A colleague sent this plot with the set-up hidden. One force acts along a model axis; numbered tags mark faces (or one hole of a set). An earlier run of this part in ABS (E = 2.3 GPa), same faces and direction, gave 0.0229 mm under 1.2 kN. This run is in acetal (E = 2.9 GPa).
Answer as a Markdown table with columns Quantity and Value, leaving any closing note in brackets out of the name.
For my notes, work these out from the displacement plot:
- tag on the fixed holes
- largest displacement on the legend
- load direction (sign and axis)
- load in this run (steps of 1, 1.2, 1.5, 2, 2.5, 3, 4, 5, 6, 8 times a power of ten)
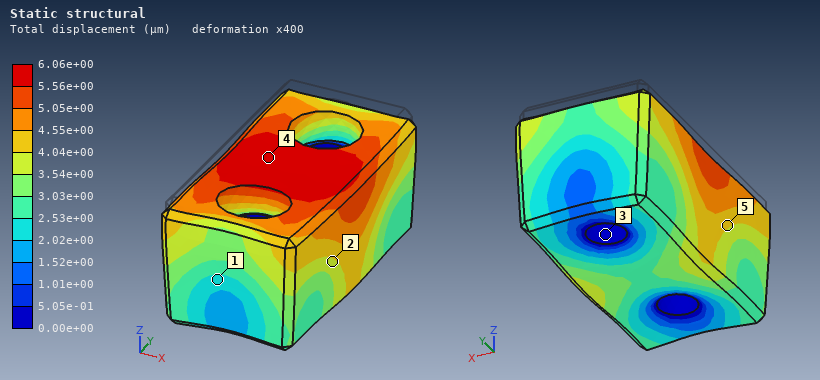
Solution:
| Quantity | Value |
|---|---|
| tag on the fixed holes | 3 |
| largest displacement on the legend | 6.06e+00 µm |
| load direction | -Z |
| load in this run | 400 N |
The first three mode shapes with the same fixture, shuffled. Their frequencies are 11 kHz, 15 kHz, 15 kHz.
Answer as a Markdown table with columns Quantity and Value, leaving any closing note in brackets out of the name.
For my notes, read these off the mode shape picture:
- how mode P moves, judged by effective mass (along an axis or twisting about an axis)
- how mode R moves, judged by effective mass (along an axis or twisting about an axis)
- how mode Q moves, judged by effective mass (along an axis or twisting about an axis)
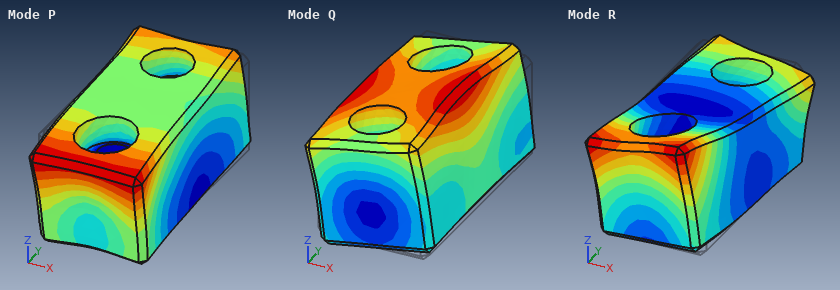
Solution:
| Quantity | Value |
|---|---|
| how mode P moves, judged by effective mass | along Y |
| how mode R moves, judged by effective mass | twisting about Z |
| how mode Q moves, judged by effective mass | along X |
